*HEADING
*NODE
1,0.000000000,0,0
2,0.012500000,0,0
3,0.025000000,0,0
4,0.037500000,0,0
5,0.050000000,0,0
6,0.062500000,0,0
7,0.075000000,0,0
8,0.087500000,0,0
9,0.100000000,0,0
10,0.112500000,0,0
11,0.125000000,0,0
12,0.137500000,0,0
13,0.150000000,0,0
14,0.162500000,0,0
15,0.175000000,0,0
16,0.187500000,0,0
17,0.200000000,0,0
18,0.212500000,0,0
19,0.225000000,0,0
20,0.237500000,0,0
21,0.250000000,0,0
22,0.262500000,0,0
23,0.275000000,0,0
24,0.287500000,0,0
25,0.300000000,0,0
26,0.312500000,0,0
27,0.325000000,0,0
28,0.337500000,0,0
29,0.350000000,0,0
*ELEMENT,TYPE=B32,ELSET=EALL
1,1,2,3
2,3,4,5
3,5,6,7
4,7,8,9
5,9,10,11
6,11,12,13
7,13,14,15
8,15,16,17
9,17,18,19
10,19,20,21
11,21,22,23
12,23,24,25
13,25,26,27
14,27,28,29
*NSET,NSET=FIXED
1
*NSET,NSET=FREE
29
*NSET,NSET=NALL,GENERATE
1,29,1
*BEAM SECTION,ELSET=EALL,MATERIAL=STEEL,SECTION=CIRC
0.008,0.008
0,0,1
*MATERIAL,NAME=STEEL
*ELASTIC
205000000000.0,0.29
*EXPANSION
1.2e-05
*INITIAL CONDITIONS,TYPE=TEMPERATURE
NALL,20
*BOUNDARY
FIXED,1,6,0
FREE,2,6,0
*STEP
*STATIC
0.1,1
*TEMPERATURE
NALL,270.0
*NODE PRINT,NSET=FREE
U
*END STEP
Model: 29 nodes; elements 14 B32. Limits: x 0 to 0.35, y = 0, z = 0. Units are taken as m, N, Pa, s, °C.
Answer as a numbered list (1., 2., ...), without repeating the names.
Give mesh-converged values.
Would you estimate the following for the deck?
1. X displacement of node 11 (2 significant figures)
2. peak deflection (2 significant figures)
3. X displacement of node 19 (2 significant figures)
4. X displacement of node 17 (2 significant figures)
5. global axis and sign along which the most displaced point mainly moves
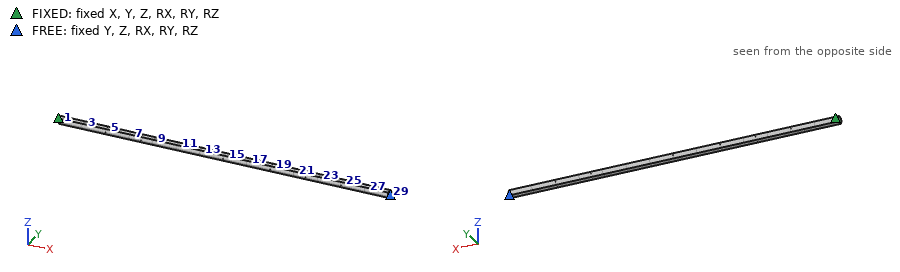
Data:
1. 3.8e-04 m
2. 0.0011 m
3. 6.8e-04 m
4. 6.0e-04 m
5. +X
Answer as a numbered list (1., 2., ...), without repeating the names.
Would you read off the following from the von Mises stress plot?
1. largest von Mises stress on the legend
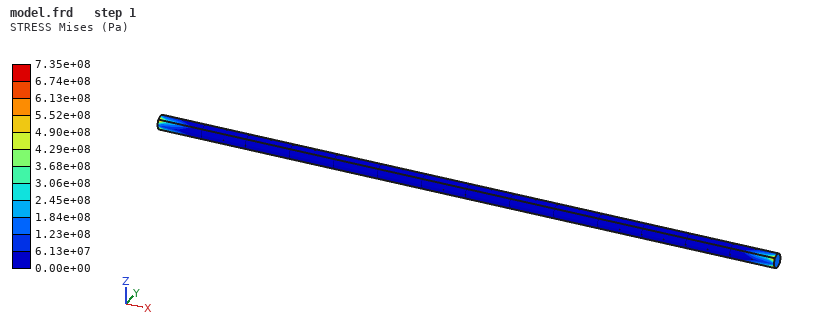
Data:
1. 7.35e+08 Pa
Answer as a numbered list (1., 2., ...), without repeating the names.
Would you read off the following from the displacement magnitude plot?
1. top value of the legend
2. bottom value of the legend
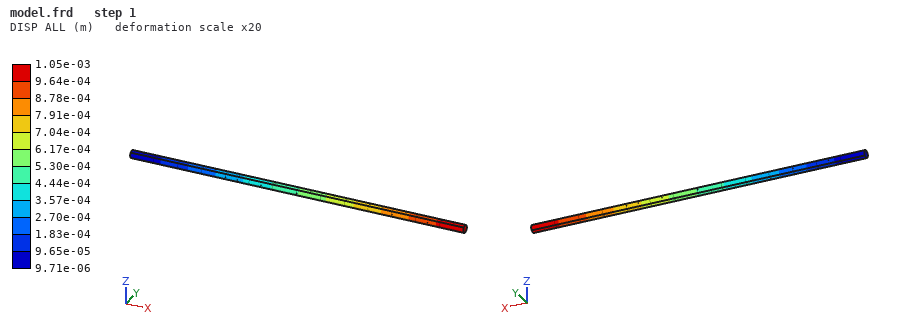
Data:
1. 1.05e-03 m
2. 9.71e-06 m
